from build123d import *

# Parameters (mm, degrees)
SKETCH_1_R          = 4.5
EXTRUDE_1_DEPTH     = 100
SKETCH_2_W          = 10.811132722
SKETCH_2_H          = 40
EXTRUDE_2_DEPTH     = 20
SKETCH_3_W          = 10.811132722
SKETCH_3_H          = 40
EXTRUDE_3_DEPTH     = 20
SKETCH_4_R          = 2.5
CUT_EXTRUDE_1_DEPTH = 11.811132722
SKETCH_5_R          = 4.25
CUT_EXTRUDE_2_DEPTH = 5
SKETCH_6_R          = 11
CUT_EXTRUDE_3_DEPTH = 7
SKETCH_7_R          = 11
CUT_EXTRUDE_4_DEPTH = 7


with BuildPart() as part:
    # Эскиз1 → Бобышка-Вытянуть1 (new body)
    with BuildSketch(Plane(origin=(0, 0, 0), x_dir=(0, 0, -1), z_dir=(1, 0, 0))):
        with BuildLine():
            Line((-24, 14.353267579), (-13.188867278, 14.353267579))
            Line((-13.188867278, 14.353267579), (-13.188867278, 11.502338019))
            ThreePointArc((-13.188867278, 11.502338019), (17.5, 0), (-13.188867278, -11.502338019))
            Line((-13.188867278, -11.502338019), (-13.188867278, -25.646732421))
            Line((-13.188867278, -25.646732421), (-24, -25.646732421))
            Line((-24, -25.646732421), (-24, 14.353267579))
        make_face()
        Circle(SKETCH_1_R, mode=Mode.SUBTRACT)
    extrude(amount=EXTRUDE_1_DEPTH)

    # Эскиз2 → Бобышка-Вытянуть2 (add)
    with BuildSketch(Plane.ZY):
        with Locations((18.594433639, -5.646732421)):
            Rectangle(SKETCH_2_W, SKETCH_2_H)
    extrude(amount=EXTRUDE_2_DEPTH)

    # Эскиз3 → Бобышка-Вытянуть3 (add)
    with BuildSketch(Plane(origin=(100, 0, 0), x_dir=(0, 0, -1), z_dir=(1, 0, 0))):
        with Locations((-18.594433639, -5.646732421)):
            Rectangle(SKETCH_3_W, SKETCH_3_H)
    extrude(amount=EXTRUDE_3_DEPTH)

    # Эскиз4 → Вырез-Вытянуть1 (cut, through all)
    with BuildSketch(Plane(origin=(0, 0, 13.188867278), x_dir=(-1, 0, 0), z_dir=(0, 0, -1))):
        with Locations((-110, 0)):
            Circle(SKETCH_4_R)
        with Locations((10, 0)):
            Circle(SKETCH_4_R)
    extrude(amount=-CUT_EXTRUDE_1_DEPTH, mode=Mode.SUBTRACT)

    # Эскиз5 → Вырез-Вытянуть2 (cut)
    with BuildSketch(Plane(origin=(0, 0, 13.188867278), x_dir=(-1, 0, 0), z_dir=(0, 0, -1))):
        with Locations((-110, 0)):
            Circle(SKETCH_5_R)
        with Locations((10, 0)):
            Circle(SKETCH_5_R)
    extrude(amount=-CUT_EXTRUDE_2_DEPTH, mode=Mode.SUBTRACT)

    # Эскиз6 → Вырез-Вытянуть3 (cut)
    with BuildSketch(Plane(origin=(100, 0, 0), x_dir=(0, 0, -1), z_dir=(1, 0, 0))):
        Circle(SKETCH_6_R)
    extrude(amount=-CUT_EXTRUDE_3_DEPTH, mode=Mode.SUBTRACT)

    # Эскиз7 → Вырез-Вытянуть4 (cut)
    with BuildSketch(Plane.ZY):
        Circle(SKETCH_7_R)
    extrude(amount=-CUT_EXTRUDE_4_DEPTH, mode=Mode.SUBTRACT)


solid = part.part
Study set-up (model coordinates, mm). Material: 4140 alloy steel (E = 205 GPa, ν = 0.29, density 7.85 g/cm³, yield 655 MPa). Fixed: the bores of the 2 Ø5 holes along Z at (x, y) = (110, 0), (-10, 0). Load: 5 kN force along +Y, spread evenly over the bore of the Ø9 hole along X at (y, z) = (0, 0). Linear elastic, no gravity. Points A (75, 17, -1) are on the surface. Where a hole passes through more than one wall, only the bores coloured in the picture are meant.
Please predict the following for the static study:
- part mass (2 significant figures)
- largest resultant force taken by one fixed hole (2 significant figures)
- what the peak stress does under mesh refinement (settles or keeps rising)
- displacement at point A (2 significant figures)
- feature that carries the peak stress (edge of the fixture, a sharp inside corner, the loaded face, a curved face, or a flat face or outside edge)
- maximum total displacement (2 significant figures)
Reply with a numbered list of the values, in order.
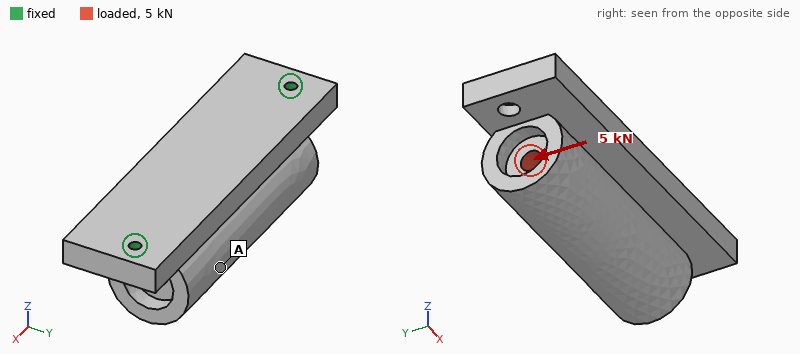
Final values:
1. 1.1 kg
2. 2.7 kN
3. keeps rising
4. 68 µm
5. edge of the fixture
6. 93 µm
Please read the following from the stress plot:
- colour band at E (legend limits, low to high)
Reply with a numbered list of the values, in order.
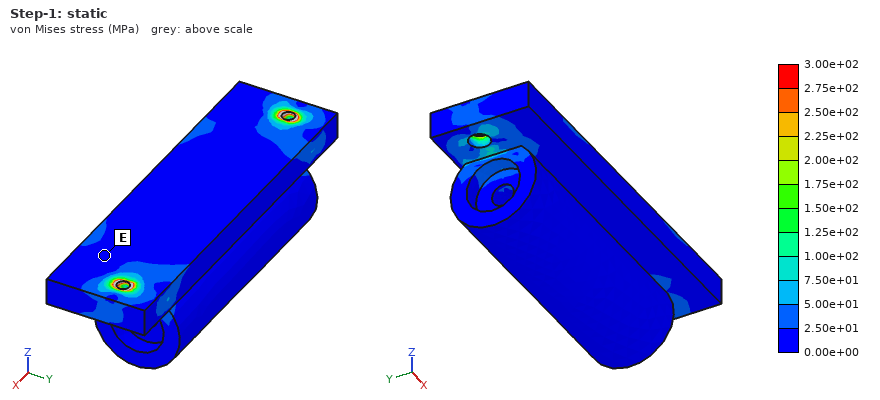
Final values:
1. 0.00e+00 to 2.50e+01 MPa
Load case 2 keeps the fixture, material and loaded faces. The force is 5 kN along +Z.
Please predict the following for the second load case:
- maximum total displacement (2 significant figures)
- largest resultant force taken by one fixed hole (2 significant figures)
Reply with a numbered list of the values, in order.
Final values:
1. 8.6 µm
2. 3.4 kN
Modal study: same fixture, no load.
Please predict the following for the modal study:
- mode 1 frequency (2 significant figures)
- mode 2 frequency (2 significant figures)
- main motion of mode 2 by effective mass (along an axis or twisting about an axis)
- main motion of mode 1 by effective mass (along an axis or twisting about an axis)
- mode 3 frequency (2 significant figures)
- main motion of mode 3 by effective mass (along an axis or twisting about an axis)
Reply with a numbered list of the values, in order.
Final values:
1. 1500 Hz
2. 4200 Hz
3. along Z
4. along Y
5. 6100 Hz
6. along Y
